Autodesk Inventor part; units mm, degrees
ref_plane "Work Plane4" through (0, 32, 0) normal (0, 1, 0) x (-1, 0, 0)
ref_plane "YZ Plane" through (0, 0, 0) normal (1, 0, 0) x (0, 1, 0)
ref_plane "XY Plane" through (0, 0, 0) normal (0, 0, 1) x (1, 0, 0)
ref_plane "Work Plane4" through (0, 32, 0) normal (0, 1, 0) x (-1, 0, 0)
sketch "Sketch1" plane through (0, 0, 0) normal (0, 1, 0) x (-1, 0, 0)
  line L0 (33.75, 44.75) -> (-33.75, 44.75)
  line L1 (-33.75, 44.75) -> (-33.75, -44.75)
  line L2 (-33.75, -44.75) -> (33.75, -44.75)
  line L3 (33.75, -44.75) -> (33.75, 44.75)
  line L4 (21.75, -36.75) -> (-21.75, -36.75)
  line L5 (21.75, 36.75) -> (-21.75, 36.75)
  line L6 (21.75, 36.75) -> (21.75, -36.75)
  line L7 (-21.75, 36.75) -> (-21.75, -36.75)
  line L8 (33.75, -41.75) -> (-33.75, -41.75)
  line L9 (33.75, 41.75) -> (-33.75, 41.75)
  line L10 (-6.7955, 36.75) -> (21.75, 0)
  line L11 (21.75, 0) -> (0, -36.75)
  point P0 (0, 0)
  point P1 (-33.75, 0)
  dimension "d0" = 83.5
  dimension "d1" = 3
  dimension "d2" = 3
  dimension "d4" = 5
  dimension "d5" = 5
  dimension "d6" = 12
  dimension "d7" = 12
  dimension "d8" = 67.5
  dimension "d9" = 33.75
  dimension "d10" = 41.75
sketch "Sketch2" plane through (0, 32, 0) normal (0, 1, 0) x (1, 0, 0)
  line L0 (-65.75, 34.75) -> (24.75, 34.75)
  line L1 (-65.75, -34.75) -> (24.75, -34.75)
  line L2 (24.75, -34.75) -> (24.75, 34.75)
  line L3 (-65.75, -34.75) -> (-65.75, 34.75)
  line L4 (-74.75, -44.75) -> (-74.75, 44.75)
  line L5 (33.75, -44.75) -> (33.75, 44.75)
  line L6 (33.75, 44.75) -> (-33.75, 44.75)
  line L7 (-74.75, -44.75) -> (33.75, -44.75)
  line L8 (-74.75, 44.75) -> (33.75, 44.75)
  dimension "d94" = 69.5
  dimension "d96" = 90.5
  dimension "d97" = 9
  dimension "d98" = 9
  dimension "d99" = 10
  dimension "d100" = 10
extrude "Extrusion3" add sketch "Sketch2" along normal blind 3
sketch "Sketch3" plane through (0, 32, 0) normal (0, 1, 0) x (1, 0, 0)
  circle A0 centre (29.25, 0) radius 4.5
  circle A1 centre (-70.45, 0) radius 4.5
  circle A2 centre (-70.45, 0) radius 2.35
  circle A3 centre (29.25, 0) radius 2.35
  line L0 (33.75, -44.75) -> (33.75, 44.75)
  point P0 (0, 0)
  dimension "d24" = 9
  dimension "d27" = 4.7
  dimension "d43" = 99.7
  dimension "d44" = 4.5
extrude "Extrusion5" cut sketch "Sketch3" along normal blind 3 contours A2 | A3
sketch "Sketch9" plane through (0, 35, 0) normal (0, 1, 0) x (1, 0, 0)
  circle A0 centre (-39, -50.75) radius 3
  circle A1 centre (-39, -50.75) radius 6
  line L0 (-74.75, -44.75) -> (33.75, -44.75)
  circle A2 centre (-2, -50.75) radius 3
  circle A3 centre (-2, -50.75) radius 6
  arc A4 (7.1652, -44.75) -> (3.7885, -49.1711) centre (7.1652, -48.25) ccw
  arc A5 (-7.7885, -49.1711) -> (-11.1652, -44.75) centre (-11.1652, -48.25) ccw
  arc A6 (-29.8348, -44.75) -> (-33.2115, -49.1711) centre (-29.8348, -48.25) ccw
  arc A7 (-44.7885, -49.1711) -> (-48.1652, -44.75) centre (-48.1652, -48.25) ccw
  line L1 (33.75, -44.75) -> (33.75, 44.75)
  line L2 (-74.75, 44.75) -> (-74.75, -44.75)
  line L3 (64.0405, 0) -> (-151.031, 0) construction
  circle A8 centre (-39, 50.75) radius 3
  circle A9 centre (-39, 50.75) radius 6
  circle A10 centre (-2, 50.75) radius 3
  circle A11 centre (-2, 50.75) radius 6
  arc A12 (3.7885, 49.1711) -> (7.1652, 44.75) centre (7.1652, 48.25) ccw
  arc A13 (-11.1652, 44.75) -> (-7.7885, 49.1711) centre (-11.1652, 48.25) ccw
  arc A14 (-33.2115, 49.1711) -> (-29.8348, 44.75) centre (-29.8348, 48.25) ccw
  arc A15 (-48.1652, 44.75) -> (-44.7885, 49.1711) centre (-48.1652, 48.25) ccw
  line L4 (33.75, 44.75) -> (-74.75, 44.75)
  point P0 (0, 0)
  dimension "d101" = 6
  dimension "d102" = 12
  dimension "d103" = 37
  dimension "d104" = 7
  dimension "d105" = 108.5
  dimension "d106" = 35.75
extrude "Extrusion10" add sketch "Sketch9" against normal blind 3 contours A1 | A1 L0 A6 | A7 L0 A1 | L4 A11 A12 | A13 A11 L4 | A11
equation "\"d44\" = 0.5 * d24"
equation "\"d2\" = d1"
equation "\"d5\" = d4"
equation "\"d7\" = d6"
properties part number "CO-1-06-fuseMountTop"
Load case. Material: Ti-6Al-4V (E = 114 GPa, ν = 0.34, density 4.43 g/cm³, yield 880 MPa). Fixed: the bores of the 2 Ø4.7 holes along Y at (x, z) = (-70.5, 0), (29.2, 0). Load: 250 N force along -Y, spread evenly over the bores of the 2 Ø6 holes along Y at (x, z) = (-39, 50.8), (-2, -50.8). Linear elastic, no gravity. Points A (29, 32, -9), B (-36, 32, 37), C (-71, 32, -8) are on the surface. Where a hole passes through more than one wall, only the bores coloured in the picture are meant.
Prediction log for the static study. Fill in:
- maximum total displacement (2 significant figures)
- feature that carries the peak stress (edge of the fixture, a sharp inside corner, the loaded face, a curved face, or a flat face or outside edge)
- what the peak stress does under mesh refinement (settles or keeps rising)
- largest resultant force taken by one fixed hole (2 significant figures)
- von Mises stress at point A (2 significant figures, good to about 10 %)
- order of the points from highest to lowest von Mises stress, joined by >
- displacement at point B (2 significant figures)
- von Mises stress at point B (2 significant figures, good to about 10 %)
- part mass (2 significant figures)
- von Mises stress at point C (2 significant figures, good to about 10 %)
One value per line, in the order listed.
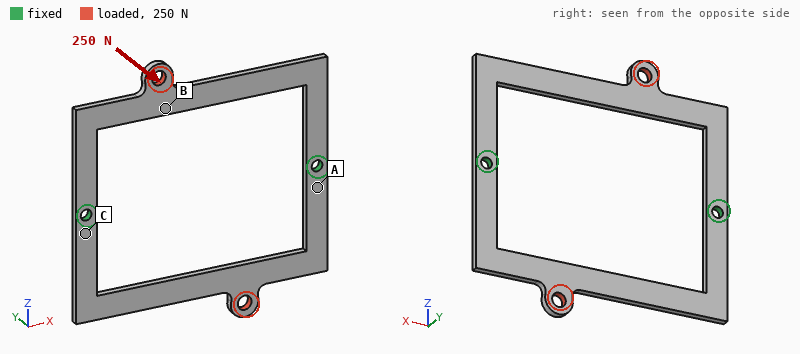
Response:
1.9 mm
edge of the fixture
keeps rising
130 N
240 MPa
A > C > B
1.1 mm
90 MPa
48 g
160 MPa
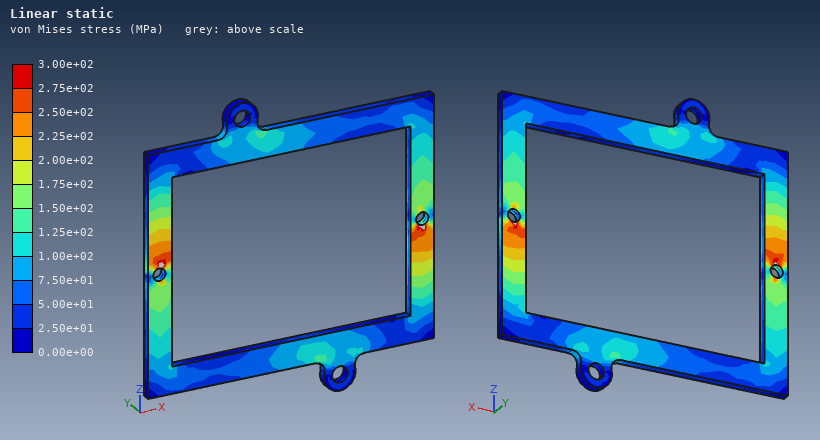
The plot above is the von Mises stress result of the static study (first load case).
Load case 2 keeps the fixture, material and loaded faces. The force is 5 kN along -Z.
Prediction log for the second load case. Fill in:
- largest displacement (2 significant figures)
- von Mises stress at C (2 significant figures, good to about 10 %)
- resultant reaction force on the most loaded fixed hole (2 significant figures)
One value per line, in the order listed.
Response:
0.56 mm
82 MPa
2.5 kN
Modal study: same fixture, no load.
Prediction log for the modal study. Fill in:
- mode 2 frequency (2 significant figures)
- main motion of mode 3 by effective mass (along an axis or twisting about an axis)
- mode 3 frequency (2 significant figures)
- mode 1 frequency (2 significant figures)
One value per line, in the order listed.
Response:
520 Hz
twisting about Z
1200 Hz
520 Hz
